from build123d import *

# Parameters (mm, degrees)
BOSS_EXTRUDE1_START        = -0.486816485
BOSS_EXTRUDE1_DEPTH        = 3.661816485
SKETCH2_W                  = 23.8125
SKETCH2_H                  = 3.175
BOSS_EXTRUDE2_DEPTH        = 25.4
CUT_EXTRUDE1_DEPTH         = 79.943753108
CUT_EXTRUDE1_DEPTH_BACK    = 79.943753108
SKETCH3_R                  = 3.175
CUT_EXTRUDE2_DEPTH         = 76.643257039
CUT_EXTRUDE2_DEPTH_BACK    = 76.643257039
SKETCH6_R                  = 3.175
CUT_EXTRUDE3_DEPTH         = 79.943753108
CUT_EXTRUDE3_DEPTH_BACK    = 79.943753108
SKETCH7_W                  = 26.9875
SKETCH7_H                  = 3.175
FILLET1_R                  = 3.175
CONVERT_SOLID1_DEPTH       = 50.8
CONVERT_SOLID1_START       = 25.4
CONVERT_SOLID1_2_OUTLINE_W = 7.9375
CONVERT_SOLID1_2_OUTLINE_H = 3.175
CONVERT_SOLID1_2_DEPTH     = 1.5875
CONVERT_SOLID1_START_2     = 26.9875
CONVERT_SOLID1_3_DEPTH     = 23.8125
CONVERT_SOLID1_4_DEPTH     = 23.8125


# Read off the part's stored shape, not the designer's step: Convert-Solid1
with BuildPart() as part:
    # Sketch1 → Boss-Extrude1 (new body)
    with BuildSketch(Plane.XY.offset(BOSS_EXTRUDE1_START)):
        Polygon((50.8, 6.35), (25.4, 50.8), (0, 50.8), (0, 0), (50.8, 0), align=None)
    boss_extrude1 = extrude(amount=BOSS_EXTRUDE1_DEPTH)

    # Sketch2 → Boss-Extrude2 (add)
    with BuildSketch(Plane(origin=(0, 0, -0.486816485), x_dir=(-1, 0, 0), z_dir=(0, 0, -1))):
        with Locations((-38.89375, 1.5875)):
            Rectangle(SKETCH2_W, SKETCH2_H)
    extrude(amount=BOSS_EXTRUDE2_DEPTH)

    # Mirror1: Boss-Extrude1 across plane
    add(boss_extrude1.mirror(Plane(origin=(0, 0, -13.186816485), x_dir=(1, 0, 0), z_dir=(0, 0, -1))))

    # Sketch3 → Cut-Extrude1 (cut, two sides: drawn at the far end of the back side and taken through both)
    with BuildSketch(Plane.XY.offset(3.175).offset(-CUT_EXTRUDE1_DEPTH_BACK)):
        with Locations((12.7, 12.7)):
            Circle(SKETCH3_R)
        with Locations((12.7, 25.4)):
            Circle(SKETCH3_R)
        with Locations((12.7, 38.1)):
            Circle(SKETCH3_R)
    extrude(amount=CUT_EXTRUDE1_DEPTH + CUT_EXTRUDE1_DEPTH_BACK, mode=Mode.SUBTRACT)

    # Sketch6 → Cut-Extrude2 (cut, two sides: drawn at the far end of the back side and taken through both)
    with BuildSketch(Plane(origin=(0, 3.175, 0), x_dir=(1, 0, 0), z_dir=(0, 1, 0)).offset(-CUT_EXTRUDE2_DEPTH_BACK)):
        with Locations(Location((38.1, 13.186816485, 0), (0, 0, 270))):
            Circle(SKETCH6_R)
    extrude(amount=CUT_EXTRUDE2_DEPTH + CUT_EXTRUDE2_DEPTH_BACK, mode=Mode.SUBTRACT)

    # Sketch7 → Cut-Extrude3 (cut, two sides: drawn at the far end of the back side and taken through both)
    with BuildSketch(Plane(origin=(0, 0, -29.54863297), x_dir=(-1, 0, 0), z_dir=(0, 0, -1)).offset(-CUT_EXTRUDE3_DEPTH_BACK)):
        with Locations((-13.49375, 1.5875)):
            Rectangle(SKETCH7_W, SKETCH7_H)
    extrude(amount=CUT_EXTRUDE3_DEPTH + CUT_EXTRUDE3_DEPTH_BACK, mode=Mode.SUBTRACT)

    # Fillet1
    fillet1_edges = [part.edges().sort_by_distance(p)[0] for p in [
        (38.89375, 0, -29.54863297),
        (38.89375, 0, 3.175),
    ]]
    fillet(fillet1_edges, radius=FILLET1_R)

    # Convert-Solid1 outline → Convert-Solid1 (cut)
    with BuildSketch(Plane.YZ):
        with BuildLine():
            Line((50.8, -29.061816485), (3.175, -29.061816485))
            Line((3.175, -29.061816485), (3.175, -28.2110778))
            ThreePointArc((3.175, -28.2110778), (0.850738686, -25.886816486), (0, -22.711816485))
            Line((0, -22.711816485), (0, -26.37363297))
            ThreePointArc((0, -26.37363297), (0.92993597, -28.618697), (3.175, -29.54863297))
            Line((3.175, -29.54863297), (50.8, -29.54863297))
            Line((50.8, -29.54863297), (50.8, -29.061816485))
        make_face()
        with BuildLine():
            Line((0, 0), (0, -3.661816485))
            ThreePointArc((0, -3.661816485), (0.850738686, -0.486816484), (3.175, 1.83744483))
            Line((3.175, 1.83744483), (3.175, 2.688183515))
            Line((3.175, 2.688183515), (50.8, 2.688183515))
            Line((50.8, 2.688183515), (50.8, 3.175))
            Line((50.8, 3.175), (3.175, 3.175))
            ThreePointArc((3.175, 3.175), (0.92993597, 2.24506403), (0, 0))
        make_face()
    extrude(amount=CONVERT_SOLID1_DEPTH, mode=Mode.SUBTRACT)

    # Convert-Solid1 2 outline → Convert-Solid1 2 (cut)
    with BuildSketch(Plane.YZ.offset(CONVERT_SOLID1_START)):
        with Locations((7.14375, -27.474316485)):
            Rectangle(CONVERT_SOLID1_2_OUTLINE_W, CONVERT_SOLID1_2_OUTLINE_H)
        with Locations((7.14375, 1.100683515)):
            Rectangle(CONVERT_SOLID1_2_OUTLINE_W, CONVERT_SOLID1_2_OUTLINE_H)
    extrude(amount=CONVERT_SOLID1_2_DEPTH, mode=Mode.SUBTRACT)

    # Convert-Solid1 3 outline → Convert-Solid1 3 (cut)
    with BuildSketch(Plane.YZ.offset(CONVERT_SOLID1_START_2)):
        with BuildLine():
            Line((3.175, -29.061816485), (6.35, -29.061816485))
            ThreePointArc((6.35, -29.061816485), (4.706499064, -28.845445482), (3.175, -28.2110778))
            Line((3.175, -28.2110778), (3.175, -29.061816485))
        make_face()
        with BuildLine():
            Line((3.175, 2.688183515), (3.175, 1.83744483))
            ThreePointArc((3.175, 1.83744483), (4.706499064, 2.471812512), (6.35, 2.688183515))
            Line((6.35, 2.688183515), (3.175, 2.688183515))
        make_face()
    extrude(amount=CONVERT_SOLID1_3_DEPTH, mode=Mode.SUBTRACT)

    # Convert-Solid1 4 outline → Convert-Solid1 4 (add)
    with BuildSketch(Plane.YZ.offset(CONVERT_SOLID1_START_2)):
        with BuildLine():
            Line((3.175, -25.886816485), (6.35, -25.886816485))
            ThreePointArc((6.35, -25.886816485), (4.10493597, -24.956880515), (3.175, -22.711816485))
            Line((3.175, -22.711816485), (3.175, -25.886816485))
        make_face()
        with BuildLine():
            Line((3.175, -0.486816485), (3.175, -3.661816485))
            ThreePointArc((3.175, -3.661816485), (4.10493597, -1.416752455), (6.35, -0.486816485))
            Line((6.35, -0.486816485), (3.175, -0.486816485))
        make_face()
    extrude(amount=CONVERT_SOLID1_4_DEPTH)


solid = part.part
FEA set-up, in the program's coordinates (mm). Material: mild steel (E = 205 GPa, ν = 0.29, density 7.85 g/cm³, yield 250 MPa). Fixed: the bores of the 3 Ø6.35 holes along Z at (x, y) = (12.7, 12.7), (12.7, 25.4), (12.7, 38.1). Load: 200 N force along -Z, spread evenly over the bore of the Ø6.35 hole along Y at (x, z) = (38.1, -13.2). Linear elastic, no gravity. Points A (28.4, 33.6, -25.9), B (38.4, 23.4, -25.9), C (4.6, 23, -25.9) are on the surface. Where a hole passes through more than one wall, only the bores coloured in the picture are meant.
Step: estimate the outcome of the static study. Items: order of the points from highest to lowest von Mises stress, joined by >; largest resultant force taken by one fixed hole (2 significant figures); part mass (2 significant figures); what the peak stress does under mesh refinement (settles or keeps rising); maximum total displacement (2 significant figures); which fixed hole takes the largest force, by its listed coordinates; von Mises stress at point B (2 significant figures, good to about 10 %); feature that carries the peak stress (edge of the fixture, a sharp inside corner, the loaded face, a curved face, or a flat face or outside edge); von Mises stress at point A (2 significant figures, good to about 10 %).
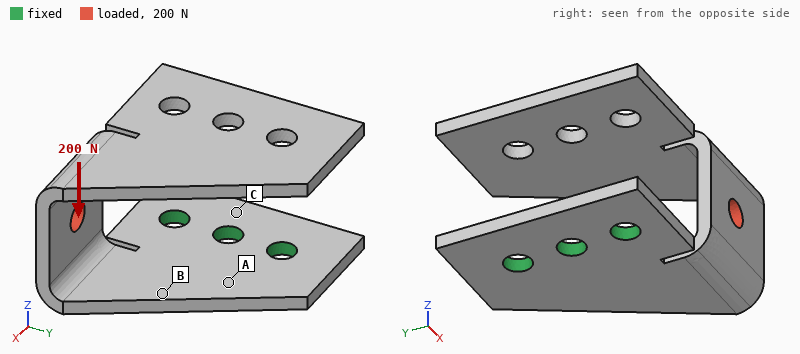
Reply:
B > A > C
270 N
100 g
keeps rising
0.33 mm
(12.7, 12.7)
67 MPa
a sharp inside corner
42 MPa
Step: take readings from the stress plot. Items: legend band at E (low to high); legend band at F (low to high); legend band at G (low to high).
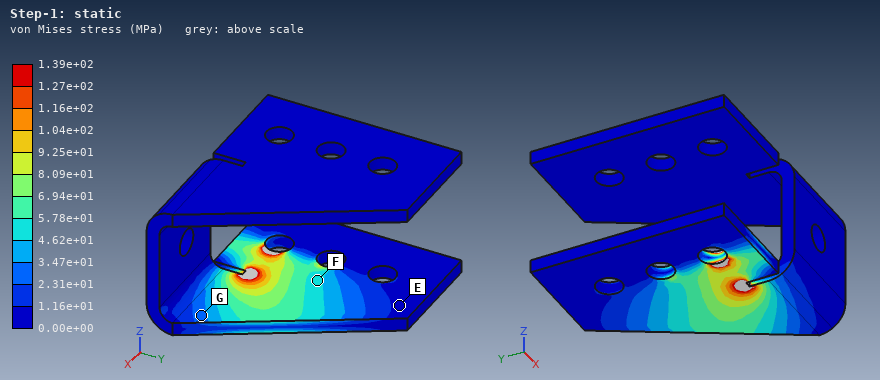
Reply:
0.00e+00 to 1.16e+01 MPa
4.62e+01 to 5.78e+01 MPa
2.31e+01 to 3.47e+01 MPa
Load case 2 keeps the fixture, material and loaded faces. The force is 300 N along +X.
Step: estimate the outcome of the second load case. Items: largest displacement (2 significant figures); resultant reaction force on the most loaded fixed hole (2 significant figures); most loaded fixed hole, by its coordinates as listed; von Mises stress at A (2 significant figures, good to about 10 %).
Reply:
0.41 mm
350 N
(12.7, 12.7)
53 MPa
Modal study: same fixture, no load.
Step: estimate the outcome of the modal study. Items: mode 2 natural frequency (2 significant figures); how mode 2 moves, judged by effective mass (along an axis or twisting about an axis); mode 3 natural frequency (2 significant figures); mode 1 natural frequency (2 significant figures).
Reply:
420 Hz
along X
770 Hz
330 Hz
